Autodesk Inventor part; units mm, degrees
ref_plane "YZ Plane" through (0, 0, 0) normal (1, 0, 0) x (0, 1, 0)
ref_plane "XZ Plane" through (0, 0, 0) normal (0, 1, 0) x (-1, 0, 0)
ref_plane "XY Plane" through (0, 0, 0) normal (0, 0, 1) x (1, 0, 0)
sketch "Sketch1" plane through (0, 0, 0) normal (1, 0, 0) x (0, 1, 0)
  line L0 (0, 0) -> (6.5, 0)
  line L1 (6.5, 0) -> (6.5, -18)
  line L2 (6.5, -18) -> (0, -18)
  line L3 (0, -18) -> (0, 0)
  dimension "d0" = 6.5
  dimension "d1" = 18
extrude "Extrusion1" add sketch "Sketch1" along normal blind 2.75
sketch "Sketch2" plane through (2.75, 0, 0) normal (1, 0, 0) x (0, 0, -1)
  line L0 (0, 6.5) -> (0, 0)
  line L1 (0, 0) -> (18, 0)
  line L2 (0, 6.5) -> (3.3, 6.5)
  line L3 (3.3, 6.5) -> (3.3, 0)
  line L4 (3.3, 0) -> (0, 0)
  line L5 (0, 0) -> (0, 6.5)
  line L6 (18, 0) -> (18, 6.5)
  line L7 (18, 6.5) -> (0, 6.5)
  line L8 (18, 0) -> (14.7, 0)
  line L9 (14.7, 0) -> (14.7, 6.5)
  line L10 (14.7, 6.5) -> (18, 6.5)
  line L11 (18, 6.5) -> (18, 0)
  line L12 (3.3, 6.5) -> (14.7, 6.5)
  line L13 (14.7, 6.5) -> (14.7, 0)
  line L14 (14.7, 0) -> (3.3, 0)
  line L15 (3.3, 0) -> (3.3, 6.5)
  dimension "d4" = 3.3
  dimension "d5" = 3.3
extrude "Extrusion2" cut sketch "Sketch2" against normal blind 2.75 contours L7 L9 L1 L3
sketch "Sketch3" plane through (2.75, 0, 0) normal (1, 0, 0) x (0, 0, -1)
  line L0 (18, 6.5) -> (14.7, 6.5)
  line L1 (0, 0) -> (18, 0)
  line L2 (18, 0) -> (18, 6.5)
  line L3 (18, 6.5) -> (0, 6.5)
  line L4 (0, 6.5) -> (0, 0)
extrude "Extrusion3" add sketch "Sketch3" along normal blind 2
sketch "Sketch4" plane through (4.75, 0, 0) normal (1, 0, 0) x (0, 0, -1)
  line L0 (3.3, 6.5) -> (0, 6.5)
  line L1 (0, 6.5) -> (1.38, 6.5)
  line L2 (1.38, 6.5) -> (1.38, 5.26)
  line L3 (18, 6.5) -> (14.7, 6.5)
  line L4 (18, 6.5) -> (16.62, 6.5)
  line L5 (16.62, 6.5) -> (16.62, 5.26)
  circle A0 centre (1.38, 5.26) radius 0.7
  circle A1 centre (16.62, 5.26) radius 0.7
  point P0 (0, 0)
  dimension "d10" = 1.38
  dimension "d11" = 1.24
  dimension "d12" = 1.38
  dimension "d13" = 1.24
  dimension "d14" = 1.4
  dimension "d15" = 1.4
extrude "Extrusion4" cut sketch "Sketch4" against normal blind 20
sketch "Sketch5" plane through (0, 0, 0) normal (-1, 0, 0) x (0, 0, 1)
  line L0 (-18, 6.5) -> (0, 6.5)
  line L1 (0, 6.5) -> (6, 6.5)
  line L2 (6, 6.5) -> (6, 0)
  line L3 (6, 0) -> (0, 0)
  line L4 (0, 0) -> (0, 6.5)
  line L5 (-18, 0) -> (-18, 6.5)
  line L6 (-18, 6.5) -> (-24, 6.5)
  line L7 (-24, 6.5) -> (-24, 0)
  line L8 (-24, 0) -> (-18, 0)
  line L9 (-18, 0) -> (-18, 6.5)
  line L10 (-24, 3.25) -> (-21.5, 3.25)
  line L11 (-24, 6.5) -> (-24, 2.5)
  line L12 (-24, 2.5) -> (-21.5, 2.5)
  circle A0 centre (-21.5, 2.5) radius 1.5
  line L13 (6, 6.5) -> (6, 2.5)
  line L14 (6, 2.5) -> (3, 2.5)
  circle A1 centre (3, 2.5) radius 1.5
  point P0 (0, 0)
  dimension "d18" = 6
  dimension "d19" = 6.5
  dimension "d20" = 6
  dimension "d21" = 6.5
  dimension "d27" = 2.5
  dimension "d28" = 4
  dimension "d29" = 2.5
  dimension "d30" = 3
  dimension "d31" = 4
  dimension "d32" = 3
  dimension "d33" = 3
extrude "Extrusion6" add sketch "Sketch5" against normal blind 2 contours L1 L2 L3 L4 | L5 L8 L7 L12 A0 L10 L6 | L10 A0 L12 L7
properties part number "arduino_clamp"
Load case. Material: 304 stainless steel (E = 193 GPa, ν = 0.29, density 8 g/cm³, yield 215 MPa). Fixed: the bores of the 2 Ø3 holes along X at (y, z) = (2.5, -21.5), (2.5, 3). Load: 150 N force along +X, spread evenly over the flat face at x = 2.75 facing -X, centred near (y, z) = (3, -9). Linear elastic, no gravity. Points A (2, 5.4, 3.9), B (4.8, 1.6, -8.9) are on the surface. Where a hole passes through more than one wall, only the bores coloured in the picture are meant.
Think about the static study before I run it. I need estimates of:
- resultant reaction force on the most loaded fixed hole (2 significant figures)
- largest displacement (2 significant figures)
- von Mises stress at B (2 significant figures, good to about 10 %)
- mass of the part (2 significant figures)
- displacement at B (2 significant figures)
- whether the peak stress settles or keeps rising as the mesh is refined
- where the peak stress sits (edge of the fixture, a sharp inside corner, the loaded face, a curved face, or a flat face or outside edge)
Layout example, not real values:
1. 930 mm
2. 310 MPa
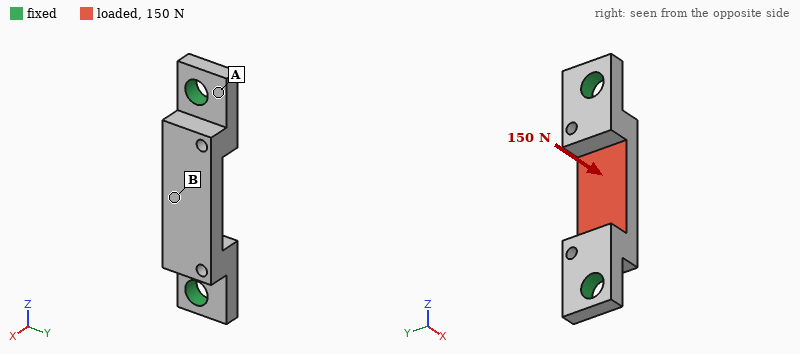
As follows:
1. 150 N
2. 3.8 µm
3. 37 MPa
4. 3.7 g
5. 3.2 µm
6. keeps rising
7. edge of the fixture
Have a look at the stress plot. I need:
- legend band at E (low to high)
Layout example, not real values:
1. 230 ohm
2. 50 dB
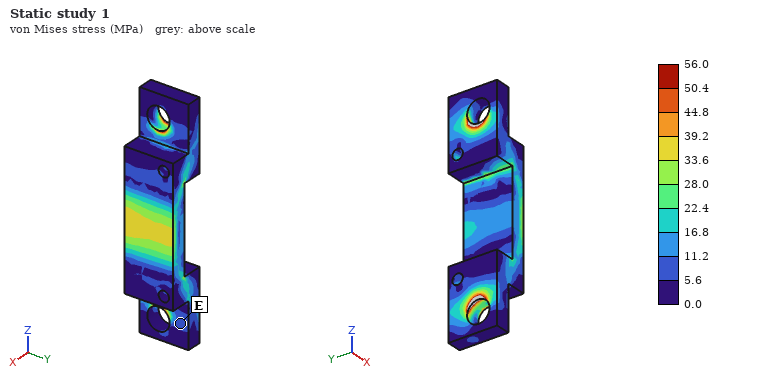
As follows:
1. 5.6 to 11.2 MPa
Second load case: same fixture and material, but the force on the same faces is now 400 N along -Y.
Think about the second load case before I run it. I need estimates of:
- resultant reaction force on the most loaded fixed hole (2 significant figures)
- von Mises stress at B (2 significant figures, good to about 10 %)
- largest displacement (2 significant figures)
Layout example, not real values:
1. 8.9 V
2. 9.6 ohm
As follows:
1. 210 N
2. 36 MPa
3. 7.3 µm
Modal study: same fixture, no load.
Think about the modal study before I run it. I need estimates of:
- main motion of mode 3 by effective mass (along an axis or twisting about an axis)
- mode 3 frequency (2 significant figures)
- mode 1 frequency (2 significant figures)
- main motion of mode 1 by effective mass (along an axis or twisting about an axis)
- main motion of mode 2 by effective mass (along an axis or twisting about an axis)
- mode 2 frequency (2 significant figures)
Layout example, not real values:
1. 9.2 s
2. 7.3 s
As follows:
1. along Z
2. 36 kHz
3. 25 kHz
4. along Y
5. along X
6. 31 kHz
